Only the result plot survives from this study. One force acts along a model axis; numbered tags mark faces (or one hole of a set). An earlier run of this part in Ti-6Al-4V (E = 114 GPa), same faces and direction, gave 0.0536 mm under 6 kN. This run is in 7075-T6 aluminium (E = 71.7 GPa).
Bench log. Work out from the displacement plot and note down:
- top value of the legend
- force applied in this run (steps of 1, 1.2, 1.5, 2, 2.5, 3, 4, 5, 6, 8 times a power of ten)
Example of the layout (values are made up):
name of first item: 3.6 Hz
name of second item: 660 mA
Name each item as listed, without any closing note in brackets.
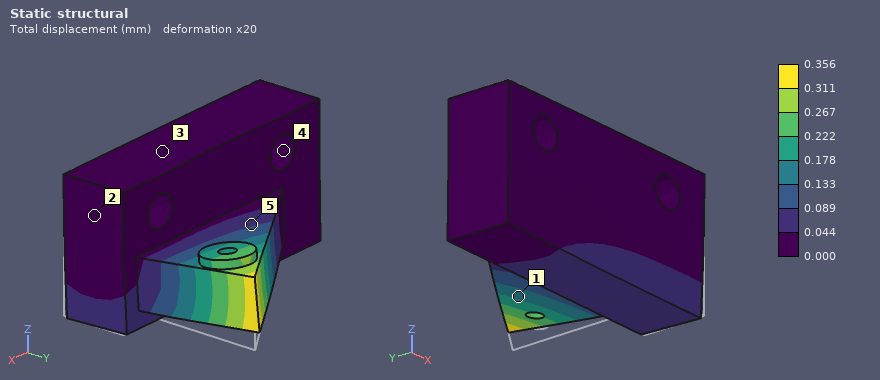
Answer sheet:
top value of the legend: 0.356 mm
force applied in this run: 25 kN
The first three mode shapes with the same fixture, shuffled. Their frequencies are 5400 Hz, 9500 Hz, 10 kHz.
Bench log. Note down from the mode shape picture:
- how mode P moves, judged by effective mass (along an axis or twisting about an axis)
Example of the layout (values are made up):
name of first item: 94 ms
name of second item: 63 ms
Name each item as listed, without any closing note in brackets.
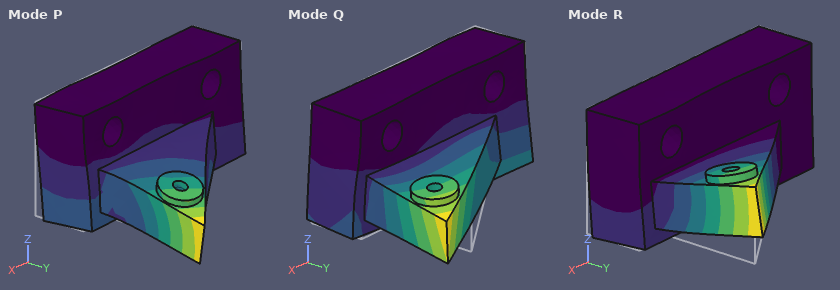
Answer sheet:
how mode P moves, judged by effective mass: along Y
